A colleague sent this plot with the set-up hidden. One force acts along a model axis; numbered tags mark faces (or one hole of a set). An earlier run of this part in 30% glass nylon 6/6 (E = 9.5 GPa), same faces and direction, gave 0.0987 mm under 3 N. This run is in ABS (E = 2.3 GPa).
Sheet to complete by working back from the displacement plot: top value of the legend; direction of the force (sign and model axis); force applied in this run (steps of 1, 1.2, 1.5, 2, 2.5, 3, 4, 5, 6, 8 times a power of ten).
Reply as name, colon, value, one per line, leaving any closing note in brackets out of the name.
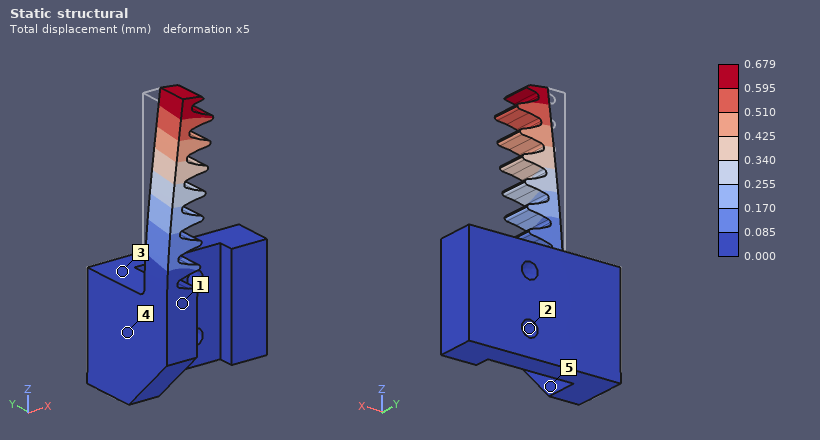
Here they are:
top value of the legend: 0.679 mm
direction of the force: +X
force applied in this run: 5 N
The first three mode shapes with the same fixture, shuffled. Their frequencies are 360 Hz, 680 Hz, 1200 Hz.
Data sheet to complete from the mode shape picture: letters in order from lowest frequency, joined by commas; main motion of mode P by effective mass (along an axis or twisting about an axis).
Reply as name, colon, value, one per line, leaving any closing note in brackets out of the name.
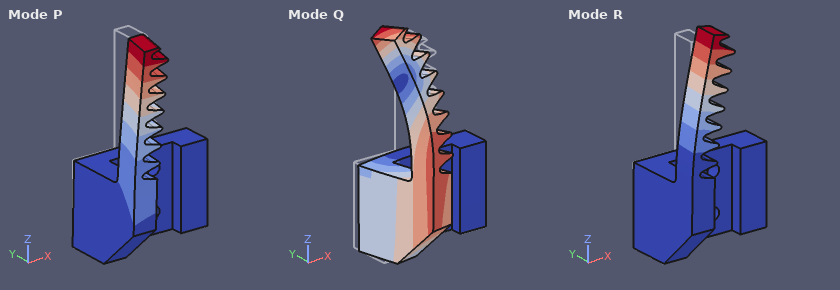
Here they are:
letters in order from lowest frequency, joined by commas: R, P, Q
main motion of mode P by effective mass: along Y
